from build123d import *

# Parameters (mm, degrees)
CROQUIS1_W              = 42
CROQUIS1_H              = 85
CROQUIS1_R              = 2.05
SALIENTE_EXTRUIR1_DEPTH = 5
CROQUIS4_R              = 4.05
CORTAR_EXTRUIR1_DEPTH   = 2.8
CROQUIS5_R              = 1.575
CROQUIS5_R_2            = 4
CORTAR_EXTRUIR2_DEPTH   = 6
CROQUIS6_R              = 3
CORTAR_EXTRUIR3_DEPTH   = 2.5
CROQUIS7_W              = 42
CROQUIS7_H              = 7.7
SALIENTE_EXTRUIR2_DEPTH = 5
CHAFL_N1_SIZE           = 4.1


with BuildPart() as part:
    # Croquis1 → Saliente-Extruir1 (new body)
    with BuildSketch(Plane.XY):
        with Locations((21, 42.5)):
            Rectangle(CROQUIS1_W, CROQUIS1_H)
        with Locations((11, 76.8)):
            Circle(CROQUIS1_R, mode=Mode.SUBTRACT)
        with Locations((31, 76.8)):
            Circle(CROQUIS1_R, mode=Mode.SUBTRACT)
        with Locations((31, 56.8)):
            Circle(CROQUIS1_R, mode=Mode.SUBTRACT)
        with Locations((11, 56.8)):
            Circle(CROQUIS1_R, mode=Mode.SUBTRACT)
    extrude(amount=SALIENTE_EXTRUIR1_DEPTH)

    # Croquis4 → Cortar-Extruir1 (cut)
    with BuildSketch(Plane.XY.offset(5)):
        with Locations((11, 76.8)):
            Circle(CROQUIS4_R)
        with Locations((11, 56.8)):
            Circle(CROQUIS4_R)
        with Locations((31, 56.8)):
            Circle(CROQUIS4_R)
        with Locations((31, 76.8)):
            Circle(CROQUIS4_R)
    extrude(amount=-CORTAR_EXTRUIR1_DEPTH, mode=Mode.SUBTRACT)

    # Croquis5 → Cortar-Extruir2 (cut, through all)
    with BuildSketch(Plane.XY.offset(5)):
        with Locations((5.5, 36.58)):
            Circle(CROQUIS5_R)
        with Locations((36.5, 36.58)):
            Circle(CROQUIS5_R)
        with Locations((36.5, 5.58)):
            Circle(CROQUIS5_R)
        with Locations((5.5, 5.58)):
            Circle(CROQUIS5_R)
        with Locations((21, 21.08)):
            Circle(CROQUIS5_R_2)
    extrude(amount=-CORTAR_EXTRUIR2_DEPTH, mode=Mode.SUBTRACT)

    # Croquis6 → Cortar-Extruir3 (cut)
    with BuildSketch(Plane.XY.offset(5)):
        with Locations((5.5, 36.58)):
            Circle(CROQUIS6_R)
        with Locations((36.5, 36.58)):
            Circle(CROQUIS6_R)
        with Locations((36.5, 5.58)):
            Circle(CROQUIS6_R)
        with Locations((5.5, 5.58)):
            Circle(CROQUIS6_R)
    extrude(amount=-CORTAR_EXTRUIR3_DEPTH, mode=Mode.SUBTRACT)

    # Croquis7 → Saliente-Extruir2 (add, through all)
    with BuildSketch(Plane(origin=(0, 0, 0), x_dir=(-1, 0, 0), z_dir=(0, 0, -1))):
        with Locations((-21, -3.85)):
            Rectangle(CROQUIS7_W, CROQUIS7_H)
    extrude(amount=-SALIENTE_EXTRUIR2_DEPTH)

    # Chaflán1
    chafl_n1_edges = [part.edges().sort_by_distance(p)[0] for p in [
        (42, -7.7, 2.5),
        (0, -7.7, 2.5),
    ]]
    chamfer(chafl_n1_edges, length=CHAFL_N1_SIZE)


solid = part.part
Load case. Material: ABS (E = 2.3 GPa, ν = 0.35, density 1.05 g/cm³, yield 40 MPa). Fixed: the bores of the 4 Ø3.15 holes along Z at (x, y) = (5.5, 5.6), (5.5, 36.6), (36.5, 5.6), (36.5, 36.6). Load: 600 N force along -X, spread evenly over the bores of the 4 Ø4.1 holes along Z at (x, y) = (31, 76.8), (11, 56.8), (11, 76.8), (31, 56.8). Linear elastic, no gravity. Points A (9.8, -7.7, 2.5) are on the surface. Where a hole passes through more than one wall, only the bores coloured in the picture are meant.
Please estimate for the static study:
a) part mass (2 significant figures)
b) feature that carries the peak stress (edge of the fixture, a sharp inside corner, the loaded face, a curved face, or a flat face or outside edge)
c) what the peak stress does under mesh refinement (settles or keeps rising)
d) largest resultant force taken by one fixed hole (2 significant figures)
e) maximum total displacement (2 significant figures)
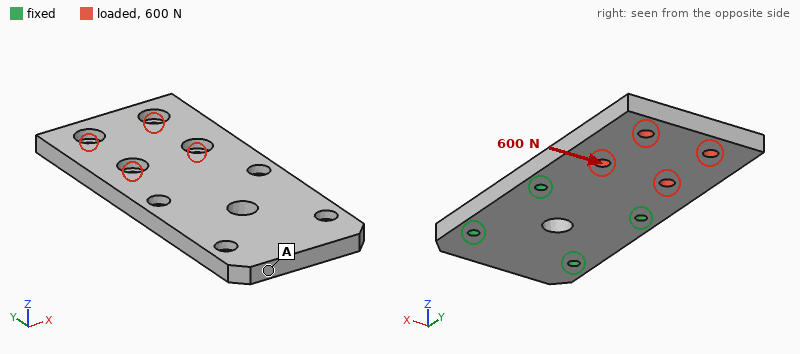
19 g
edge of the fixture
keeps rising
550 N
0.62 mm
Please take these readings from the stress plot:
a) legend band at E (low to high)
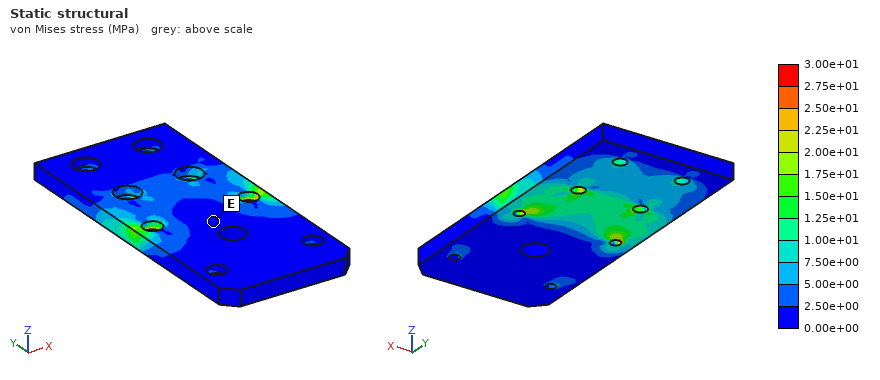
0.00e+00 to 2.50e+00 MPa
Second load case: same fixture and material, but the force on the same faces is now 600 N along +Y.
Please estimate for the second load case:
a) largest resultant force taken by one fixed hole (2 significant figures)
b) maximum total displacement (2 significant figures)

250 N
0.84 mm
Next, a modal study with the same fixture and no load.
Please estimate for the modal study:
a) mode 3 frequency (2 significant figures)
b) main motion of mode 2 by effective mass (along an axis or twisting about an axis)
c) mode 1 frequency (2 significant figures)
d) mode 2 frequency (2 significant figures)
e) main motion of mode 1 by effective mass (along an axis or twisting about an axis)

2500 Hz
twisting about Y
430 Hz
1200 Hz
along Z
